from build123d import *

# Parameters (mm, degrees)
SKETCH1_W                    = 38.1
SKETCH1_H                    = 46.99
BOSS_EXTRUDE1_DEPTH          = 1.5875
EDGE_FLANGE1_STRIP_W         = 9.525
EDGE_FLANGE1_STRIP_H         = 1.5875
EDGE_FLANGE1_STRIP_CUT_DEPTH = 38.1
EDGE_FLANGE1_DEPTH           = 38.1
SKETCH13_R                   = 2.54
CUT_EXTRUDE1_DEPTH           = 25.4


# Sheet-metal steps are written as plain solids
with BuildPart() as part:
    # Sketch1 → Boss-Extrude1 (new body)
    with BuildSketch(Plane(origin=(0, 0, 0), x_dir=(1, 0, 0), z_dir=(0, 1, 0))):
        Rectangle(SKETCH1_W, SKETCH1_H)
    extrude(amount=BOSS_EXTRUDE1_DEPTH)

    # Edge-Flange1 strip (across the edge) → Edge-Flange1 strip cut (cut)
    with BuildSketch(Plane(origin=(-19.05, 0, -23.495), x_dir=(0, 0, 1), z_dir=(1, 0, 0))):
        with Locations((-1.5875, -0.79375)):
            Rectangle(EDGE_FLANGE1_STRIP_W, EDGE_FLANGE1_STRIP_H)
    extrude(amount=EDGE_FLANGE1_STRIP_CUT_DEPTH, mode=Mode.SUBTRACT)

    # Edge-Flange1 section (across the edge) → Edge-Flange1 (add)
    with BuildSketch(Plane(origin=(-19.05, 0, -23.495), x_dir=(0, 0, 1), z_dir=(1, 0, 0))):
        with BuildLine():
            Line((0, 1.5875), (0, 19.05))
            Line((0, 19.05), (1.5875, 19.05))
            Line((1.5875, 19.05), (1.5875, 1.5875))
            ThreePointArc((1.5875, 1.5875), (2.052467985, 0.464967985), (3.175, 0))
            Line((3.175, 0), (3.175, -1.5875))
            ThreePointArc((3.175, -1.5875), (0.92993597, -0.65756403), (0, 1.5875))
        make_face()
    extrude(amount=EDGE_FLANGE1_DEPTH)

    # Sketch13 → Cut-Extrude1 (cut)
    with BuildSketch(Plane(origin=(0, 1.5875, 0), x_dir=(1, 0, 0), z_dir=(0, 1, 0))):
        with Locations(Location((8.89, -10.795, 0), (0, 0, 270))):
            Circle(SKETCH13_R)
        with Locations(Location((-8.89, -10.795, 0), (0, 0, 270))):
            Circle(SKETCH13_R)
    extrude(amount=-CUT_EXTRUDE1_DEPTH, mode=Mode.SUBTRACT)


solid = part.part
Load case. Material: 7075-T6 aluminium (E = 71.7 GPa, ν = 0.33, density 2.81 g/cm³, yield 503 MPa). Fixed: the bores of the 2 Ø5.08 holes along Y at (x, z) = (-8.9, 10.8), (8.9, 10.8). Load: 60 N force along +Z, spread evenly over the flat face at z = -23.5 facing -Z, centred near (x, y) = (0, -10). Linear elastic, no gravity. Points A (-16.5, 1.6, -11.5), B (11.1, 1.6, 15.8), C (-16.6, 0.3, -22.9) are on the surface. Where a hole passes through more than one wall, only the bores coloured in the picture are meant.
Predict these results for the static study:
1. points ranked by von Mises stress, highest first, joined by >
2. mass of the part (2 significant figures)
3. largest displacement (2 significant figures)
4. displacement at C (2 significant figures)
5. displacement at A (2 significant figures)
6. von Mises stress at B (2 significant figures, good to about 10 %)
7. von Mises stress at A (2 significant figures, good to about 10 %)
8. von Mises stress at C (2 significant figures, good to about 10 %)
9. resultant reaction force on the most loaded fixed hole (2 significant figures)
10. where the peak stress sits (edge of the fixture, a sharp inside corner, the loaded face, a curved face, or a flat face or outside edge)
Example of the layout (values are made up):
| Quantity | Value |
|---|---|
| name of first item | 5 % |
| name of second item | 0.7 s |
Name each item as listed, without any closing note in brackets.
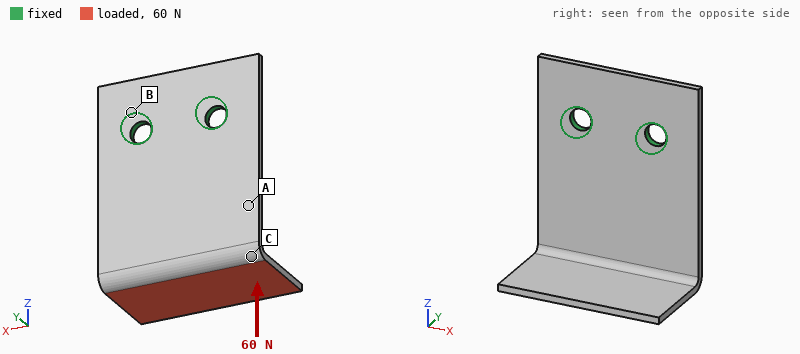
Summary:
| Quantity | Value |
|---|---|
| points ranked by von Mises stress, highest first, joined by > | A > C > B |
| mass of the part | 11 g |
| largest displacement | 0.62 mm |
| displacement at C | 0.36 mm |
| displacement at A | 0.15 mm |
| von Mises stress at B | 6.4 MPa |
| von Mises stress at A | 41 MPa |
| von Mises stress at C | 22 MPa |
| resultant reaction force on the most loaded fixed hole | 30 N |
| where the peak stress sits | a flat face or outside edge |
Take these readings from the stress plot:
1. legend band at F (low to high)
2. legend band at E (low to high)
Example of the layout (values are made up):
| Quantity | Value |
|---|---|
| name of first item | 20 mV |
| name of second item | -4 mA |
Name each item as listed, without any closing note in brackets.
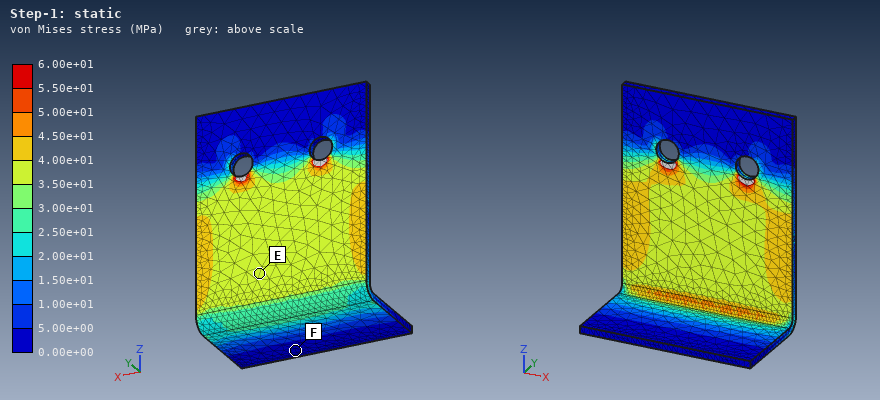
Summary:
| Quantity | Value |
|---|---|
| legend band at F | 0.00e+00 to 5.00e+00 MPa |
| legend band at E | 3.50e+01 to 4.00e+01 MPa |
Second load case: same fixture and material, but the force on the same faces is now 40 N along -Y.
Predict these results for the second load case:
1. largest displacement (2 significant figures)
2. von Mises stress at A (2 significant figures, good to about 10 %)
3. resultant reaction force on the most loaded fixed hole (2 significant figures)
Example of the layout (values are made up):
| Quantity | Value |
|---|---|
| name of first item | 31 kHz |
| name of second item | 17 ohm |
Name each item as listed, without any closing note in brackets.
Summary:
| Quantity | Value |
|---|---|
| largest displacement | 0.67 mm |
| von Mises stress at A | 31 MPa |
| resultant reaction force on the most loaded fixed hole | 20 N |
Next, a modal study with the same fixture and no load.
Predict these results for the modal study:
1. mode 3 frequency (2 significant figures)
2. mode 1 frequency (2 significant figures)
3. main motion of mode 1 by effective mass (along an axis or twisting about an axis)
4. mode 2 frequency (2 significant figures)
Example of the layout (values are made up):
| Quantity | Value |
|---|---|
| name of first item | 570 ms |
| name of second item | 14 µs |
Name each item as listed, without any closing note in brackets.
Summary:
| Quantity | Value |
|---|---|
| mode 3 frequency | 2200 Hz |
| mode 1 frequency | 630 Hz |
| main motion of mode 1 by effective mass | along Y |
| mode 2 frequency | 1300 Hz |
